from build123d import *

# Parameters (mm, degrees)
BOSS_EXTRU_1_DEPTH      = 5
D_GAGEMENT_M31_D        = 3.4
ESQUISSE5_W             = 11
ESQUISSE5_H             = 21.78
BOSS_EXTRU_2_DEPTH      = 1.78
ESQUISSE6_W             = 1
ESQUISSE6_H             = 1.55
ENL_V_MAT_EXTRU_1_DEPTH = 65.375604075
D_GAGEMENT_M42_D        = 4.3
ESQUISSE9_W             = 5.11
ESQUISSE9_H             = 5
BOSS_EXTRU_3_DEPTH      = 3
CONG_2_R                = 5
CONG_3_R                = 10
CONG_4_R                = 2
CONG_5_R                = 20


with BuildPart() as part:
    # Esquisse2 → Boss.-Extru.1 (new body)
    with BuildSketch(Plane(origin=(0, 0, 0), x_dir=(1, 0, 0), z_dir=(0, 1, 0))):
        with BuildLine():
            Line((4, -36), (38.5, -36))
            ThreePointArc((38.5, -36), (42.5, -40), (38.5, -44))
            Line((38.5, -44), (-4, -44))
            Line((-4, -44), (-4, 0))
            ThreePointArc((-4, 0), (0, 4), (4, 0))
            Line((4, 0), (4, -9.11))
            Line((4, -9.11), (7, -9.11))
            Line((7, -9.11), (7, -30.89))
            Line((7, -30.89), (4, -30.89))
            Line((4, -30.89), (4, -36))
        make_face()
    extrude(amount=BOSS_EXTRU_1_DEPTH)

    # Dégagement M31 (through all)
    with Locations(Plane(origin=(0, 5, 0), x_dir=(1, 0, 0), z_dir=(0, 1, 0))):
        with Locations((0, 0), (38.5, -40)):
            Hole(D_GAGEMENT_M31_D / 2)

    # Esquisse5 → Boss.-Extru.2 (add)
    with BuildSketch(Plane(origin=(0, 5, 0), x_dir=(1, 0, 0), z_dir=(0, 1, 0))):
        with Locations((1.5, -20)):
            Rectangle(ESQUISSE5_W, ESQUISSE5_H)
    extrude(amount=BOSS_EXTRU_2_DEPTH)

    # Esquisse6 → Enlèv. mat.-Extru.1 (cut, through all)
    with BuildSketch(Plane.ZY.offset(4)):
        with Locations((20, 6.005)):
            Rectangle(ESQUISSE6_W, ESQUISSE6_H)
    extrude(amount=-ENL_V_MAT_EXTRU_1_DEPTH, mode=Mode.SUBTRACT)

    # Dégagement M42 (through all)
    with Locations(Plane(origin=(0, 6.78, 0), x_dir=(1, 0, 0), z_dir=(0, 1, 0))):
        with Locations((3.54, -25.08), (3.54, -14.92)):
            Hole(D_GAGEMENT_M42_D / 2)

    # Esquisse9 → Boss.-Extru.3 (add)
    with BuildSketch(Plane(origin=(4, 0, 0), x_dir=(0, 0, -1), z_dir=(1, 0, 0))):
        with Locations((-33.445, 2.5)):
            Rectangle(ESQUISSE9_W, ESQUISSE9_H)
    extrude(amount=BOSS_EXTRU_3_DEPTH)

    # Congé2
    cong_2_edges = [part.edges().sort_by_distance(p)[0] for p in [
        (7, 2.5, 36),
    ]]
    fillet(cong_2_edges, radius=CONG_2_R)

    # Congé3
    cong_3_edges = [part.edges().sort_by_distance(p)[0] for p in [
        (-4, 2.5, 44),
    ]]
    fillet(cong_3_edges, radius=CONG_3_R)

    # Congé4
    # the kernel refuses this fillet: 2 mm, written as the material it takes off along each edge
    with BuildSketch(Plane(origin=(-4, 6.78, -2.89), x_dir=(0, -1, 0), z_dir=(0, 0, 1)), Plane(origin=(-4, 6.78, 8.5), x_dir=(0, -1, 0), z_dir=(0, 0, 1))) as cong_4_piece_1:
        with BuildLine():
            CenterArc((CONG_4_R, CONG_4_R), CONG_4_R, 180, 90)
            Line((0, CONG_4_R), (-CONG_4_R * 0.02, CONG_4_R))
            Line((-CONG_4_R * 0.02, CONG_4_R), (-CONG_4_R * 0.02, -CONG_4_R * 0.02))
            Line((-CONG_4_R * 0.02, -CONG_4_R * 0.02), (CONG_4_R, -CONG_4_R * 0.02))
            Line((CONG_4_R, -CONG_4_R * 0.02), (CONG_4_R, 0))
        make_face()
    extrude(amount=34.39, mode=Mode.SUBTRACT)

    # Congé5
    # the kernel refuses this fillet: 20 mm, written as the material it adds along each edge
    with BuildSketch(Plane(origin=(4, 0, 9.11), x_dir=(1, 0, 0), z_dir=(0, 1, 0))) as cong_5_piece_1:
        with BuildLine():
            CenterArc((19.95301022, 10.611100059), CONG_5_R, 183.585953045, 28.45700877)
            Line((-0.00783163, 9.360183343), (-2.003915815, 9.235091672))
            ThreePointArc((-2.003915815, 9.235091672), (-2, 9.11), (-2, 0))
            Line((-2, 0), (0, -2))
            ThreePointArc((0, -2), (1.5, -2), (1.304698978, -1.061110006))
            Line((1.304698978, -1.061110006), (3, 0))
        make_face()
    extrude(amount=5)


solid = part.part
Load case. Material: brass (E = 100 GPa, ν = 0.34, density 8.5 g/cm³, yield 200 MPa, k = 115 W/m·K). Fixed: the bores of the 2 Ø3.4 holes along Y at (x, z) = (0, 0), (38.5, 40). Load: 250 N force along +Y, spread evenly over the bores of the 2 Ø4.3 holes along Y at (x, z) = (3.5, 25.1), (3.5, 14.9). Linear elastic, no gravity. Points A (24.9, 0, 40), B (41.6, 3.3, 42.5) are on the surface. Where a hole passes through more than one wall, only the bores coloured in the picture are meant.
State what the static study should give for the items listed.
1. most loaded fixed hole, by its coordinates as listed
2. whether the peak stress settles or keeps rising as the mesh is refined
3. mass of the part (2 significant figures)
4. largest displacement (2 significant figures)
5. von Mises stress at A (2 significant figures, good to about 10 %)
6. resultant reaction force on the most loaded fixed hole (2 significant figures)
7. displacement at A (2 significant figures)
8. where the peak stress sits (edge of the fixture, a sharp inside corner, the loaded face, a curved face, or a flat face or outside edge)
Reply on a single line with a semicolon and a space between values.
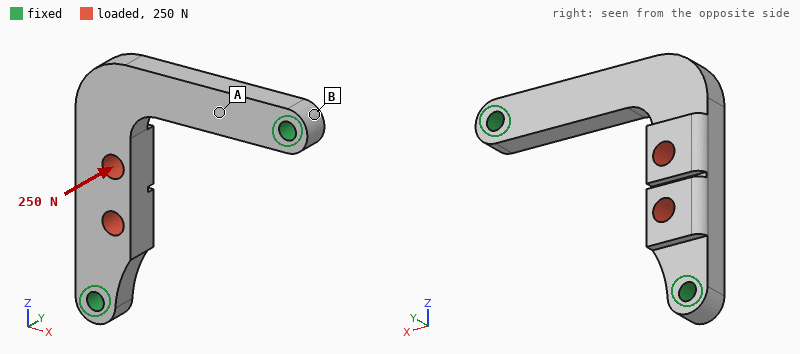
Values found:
(0, 0); keeps rising; 33 g; 50 µm; 16 MPa; 190 N; 11 µm; edge of the fixture
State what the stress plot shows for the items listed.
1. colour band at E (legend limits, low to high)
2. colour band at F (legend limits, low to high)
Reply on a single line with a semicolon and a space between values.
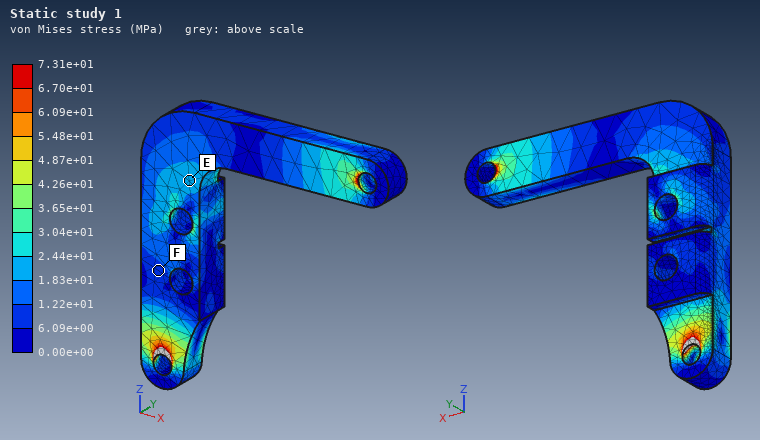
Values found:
1.83e+01 to 2.44e+01 MPa; 6.09e+00 to 1.22e+01 MPa
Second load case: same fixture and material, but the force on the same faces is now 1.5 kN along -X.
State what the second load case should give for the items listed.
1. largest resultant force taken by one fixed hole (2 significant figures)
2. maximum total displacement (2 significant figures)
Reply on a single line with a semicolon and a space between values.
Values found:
800 N; 31 µm
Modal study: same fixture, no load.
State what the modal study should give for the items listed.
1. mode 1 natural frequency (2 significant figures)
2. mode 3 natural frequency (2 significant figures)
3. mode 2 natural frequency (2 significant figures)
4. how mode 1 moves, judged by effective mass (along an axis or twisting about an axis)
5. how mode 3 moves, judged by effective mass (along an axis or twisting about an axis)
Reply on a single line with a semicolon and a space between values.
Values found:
2300 Hz; 10 kHz; 8300 Hz; along Y; along X
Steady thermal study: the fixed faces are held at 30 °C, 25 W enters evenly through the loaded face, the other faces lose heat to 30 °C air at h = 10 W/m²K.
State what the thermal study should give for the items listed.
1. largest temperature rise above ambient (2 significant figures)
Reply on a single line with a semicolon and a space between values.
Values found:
58 K
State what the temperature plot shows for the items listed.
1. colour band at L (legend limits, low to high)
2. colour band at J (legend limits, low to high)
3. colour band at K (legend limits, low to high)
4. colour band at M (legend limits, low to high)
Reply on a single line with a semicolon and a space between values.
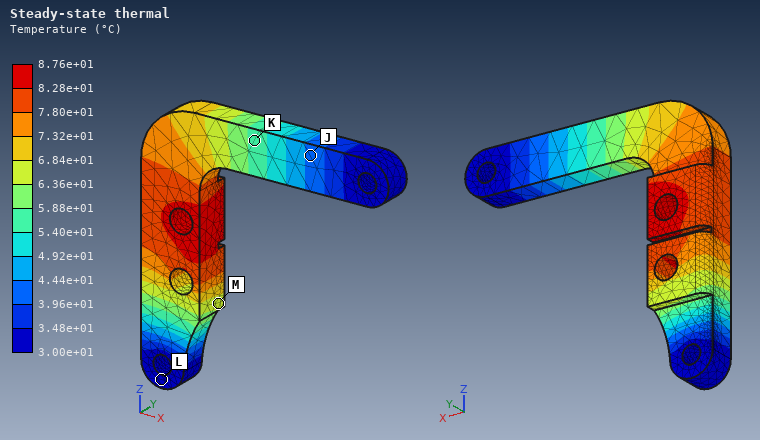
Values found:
3.00e+01 to 3.48e+01 °C; 3.96e+01 to 4.44e+01 °C; 5.40e+01 to 5.88e+01 °C; 6.36e+01 to 6.84e+01 °C
